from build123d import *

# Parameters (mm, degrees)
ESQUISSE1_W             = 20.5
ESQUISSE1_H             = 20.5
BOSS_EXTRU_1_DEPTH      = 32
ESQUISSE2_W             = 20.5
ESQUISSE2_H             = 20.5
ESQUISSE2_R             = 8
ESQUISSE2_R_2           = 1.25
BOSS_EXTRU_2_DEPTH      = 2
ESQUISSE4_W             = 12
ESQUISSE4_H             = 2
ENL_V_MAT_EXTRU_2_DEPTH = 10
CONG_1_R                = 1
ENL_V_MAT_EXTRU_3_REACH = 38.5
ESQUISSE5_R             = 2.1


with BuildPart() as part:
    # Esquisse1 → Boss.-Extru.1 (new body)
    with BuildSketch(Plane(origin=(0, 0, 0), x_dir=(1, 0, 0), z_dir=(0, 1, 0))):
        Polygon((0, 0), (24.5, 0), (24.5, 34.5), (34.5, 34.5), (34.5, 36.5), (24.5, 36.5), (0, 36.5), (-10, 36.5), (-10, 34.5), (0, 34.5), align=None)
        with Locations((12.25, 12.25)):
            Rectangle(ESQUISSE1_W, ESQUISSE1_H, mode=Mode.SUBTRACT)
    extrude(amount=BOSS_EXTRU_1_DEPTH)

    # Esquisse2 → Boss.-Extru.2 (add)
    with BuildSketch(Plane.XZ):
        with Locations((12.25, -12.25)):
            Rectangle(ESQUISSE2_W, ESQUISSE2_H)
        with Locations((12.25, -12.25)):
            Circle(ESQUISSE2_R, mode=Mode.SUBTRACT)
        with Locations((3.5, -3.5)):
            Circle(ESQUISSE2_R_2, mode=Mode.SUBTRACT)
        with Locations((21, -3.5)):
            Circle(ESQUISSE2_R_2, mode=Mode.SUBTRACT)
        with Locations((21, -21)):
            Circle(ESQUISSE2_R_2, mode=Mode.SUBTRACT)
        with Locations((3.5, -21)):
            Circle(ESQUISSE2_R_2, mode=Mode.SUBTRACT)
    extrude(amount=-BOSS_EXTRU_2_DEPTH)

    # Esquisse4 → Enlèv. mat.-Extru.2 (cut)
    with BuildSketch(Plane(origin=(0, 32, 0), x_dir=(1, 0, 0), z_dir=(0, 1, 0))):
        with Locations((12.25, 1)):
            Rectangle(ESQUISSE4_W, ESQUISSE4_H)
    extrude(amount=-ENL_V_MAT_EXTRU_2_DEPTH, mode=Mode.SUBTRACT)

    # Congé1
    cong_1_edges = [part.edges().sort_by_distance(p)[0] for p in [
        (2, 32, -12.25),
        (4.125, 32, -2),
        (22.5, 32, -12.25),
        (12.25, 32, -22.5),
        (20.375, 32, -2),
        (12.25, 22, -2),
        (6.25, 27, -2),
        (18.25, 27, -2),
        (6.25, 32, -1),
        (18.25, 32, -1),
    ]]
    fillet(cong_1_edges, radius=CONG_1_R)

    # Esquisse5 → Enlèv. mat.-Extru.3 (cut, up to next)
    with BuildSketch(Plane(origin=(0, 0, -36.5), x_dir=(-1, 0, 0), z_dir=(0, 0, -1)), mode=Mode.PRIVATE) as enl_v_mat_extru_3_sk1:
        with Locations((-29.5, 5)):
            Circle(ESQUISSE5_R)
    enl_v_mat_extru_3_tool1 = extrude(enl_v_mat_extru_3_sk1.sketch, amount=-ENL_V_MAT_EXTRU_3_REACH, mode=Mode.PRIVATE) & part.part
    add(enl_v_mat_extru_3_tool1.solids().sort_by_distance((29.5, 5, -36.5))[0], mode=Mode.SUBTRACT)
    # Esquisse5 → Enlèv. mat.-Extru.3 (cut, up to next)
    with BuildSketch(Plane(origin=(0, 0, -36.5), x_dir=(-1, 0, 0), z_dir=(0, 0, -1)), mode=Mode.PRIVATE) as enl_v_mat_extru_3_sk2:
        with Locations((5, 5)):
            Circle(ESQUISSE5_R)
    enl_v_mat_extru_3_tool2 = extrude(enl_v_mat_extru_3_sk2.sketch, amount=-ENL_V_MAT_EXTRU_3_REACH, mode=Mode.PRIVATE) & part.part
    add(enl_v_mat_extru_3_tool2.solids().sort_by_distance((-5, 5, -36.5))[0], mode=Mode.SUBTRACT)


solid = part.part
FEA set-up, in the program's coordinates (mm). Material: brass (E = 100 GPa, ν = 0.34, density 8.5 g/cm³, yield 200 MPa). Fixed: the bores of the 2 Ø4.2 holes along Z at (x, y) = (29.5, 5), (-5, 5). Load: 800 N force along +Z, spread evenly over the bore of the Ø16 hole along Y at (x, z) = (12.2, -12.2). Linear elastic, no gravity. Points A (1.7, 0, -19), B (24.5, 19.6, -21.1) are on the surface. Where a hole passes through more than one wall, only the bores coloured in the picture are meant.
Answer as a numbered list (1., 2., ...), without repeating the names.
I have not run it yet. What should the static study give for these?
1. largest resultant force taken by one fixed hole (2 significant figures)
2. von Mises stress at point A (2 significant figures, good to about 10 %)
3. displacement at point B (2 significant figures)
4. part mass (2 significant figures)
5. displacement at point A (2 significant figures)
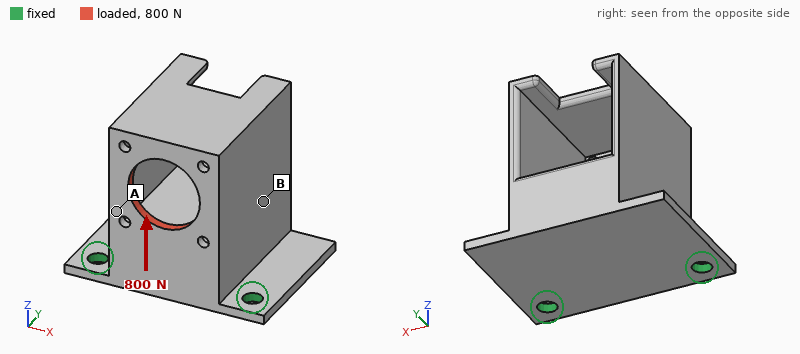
1. 450 N
2. 23 MPa
3. 0.060 mm
4. 140 g
5. 0.061 mm
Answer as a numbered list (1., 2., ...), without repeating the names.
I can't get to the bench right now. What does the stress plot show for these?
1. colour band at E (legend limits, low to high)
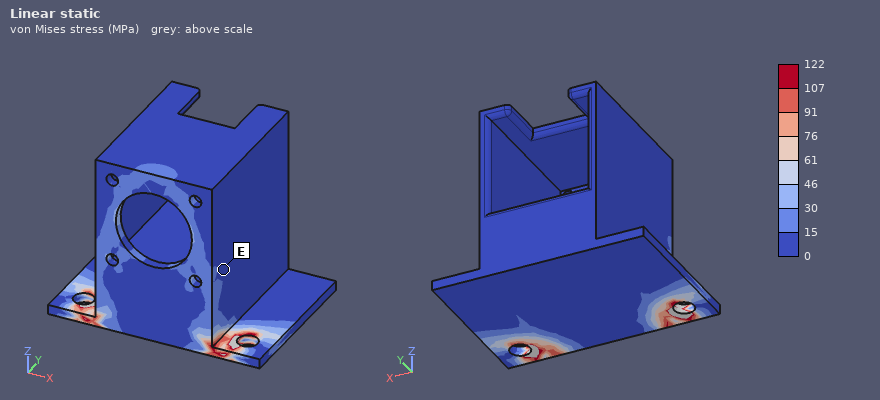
1. 0 to 15 MPa
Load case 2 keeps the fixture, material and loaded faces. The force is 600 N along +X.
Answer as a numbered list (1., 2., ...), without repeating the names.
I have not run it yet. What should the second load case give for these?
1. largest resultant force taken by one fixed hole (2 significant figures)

1. 580 N
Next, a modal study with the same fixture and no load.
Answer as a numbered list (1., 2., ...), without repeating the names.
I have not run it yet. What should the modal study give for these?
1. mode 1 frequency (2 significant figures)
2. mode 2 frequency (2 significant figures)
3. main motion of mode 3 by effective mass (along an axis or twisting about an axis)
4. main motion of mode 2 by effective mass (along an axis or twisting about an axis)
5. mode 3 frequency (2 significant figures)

1. 690 Hz
2. 2600 Hz
3. along Z
4. along X
5. 4800 Hz
